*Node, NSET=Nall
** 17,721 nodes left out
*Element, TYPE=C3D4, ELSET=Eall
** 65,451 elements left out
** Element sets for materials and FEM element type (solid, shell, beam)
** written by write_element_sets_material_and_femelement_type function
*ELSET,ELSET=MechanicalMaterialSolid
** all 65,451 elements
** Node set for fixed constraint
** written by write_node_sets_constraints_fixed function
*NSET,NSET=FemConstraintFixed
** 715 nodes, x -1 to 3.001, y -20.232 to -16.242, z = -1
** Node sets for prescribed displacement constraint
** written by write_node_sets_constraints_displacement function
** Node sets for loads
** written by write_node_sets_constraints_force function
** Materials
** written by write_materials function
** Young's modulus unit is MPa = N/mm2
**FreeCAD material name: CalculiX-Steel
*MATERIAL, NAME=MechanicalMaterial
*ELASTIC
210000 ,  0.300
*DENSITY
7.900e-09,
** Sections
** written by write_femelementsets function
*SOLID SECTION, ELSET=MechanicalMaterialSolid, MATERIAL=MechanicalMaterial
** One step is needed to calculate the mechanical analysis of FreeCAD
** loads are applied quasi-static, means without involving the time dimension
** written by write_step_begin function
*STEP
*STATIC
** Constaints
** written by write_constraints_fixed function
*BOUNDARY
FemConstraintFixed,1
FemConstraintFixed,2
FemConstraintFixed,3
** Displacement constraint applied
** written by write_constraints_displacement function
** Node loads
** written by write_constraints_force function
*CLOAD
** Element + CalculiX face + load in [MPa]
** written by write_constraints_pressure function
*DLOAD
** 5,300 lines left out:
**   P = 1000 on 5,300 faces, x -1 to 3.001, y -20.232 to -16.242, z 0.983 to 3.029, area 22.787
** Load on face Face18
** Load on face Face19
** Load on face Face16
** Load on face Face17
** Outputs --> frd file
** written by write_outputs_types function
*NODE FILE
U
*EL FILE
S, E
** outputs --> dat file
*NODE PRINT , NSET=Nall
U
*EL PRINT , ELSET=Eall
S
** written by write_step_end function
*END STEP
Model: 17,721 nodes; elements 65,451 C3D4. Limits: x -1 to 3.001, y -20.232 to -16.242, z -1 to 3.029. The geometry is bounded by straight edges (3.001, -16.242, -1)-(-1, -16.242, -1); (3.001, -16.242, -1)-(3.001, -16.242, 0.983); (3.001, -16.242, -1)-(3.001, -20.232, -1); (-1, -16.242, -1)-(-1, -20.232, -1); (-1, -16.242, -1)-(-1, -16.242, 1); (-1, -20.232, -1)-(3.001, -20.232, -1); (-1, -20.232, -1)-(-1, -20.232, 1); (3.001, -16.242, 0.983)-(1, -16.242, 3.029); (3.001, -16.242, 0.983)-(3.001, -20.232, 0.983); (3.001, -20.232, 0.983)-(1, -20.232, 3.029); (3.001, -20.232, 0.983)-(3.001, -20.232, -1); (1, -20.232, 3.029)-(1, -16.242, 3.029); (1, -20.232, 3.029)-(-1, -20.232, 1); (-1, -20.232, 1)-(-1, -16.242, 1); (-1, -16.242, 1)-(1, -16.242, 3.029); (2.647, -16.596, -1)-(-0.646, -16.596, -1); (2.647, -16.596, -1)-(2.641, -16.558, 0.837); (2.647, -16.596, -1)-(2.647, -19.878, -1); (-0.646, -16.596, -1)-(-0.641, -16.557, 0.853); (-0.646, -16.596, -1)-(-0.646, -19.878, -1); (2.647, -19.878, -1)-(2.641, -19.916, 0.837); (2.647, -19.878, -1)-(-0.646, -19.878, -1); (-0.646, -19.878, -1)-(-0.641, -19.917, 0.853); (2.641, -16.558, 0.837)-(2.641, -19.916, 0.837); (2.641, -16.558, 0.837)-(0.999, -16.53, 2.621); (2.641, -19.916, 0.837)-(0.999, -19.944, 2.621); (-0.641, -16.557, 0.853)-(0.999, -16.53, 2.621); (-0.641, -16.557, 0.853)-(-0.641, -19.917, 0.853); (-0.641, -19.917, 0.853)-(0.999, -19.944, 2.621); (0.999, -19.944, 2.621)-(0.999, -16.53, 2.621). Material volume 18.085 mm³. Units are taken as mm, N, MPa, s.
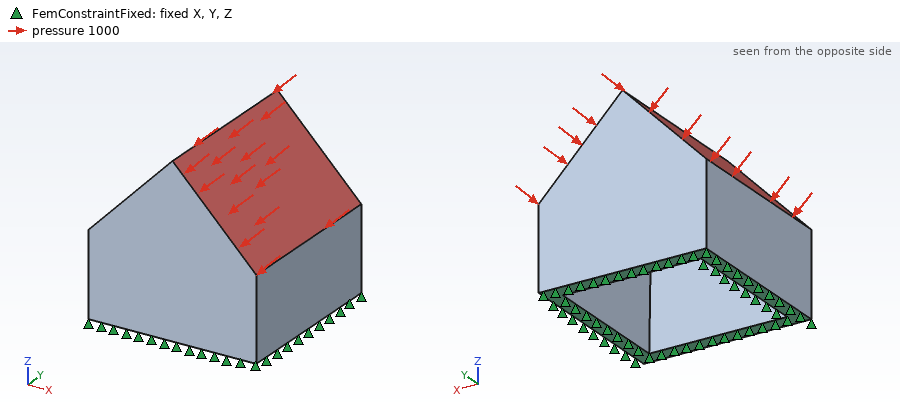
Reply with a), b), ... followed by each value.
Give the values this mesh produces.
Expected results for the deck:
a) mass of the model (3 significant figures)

a) 1.43e-04 kg
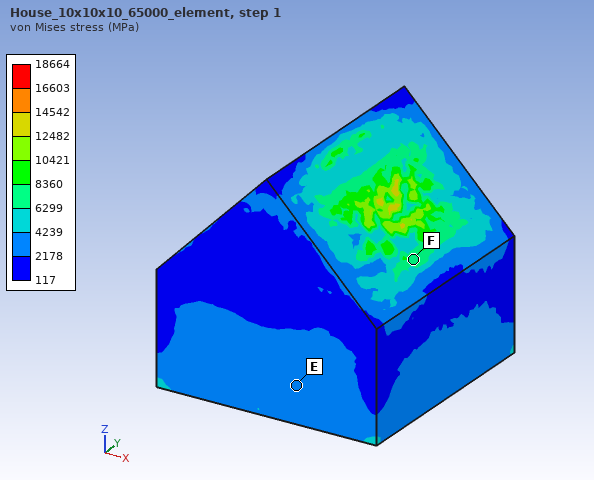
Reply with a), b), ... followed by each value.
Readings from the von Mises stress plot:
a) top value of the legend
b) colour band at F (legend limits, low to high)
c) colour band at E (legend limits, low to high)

a) 18664 MPa
b) 6299 to 8360 MPa
c) 2178 to 4239 MPa
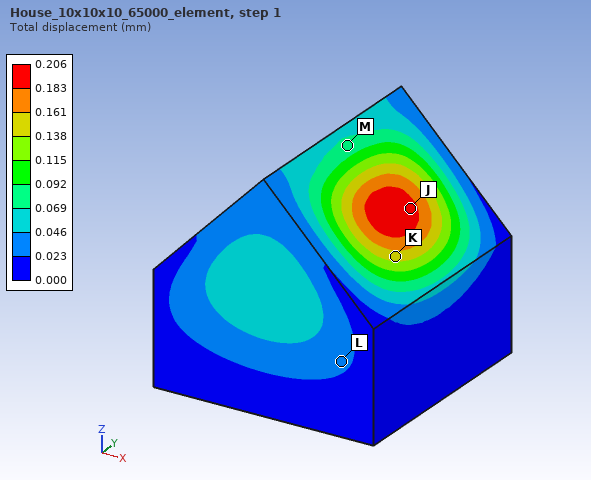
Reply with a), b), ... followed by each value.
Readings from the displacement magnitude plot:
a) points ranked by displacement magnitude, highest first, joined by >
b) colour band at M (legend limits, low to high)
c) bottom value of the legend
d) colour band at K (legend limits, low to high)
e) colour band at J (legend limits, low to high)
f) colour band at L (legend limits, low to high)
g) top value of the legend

a) J > K > M > L
b) 0.069 to 0.092 mm
c) 0.000 mm
d) 0.138 to 0.161 mm
e) 0.183 to 0.206 mm
f) 0.023 to 0.046 mm
g) 0.206 mm
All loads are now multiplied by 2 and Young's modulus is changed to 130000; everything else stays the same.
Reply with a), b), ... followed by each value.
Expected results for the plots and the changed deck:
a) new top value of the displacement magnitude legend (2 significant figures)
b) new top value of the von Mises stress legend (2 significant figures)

a) 0.67 mm
b) 37000 MPa
